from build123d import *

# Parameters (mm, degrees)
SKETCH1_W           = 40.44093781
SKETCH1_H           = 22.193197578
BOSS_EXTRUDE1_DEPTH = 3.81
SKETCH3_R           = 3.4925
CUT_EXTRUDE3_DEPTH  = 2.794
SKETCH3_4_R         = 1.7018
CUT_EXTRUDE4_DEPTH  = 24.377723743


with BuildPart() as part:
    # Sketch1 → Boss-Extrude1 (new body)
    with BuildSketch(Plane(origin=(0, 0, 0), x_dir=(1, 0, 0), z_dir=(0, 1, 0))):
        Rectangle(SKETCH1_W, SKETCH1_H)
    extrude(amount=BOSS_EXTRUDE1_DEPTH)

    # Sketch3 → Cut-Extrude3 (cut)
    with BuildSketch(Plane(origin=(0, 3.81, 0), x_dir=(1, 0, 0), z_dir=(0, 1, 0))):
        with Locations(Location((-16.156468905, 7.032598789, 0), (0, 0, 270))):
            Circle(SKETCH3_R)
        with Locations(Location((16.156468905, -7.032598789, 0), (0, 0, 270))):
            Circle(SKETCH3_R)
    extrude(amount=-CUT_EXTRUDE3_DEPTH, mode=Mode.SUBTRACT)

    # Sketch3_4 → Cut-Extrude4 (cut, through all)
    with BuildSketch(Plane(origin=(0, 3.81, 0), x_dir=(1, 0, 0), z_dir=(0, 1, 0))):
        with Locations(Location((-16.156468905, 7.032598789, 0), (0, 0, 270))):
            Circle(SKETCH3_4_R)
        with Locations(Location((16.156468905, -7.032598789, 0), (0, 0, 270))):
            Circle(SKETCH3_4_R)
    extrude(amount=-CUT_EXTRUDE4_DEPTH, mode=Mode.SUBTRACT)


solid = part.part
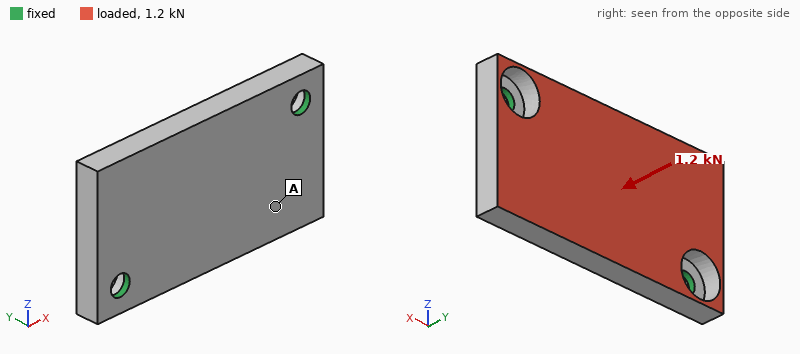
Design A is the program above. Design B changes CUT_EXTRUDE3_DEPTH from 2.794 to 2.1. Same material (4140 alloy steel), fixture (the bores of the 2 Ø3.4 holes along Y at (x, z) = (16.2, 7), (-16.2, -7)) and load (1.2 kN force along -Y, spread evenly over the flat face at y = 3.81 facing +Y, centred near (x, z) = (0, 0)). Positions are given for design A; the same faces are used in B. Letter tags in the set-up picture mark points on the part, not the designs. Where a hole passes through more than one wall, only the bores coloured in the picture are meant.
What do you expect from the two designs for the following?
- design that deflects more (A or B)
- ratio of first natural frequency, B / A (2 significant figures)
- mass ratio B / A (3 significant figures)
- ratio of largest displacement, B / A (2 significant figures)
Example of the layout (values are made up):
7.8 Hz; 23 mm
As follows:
A; 1.4; 1.01; 0.83
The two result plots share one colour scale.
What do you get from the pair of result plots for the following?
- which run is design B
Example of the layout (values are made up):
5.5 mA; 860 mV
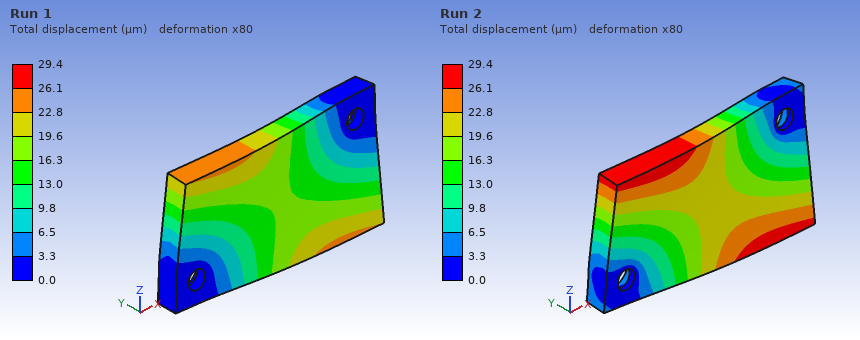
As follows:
Run 1
